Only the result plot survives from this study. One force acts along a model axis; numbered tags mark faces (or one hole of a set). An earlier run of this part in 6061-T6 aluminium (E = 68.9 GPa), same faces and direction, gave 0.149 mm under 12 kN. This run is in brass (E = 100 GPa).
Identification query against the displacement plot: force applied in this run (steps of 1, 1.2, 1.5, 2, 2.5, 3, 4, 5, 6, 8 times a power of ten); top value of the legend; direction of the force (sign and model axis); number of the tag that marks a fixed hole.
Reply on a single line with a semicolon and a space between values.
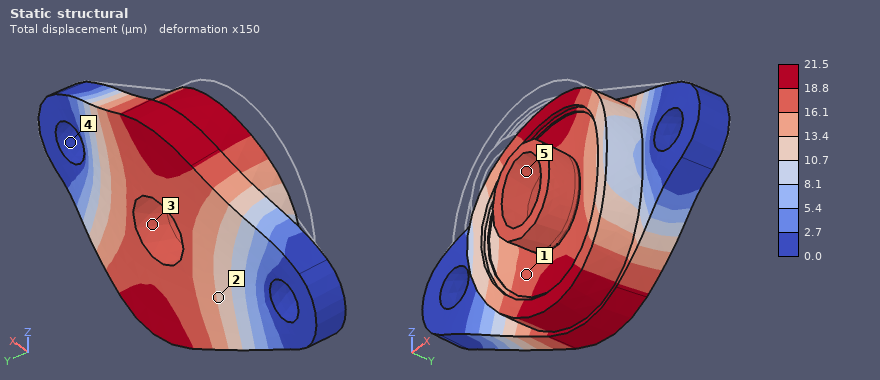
2.5 kN; 21.5 µm; +Y; 4
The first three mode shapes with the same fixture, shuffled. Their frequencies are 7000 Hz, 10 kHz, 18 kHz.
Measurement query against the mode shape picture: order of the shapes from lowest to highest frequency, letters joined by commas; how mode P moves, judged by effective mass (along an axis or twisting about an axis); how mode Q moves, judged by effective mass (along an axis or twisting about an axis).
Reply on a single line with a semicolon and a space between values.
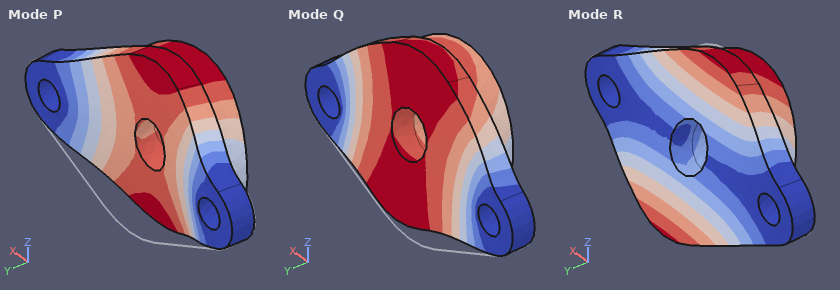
R, P, Q; along Y; along Z
